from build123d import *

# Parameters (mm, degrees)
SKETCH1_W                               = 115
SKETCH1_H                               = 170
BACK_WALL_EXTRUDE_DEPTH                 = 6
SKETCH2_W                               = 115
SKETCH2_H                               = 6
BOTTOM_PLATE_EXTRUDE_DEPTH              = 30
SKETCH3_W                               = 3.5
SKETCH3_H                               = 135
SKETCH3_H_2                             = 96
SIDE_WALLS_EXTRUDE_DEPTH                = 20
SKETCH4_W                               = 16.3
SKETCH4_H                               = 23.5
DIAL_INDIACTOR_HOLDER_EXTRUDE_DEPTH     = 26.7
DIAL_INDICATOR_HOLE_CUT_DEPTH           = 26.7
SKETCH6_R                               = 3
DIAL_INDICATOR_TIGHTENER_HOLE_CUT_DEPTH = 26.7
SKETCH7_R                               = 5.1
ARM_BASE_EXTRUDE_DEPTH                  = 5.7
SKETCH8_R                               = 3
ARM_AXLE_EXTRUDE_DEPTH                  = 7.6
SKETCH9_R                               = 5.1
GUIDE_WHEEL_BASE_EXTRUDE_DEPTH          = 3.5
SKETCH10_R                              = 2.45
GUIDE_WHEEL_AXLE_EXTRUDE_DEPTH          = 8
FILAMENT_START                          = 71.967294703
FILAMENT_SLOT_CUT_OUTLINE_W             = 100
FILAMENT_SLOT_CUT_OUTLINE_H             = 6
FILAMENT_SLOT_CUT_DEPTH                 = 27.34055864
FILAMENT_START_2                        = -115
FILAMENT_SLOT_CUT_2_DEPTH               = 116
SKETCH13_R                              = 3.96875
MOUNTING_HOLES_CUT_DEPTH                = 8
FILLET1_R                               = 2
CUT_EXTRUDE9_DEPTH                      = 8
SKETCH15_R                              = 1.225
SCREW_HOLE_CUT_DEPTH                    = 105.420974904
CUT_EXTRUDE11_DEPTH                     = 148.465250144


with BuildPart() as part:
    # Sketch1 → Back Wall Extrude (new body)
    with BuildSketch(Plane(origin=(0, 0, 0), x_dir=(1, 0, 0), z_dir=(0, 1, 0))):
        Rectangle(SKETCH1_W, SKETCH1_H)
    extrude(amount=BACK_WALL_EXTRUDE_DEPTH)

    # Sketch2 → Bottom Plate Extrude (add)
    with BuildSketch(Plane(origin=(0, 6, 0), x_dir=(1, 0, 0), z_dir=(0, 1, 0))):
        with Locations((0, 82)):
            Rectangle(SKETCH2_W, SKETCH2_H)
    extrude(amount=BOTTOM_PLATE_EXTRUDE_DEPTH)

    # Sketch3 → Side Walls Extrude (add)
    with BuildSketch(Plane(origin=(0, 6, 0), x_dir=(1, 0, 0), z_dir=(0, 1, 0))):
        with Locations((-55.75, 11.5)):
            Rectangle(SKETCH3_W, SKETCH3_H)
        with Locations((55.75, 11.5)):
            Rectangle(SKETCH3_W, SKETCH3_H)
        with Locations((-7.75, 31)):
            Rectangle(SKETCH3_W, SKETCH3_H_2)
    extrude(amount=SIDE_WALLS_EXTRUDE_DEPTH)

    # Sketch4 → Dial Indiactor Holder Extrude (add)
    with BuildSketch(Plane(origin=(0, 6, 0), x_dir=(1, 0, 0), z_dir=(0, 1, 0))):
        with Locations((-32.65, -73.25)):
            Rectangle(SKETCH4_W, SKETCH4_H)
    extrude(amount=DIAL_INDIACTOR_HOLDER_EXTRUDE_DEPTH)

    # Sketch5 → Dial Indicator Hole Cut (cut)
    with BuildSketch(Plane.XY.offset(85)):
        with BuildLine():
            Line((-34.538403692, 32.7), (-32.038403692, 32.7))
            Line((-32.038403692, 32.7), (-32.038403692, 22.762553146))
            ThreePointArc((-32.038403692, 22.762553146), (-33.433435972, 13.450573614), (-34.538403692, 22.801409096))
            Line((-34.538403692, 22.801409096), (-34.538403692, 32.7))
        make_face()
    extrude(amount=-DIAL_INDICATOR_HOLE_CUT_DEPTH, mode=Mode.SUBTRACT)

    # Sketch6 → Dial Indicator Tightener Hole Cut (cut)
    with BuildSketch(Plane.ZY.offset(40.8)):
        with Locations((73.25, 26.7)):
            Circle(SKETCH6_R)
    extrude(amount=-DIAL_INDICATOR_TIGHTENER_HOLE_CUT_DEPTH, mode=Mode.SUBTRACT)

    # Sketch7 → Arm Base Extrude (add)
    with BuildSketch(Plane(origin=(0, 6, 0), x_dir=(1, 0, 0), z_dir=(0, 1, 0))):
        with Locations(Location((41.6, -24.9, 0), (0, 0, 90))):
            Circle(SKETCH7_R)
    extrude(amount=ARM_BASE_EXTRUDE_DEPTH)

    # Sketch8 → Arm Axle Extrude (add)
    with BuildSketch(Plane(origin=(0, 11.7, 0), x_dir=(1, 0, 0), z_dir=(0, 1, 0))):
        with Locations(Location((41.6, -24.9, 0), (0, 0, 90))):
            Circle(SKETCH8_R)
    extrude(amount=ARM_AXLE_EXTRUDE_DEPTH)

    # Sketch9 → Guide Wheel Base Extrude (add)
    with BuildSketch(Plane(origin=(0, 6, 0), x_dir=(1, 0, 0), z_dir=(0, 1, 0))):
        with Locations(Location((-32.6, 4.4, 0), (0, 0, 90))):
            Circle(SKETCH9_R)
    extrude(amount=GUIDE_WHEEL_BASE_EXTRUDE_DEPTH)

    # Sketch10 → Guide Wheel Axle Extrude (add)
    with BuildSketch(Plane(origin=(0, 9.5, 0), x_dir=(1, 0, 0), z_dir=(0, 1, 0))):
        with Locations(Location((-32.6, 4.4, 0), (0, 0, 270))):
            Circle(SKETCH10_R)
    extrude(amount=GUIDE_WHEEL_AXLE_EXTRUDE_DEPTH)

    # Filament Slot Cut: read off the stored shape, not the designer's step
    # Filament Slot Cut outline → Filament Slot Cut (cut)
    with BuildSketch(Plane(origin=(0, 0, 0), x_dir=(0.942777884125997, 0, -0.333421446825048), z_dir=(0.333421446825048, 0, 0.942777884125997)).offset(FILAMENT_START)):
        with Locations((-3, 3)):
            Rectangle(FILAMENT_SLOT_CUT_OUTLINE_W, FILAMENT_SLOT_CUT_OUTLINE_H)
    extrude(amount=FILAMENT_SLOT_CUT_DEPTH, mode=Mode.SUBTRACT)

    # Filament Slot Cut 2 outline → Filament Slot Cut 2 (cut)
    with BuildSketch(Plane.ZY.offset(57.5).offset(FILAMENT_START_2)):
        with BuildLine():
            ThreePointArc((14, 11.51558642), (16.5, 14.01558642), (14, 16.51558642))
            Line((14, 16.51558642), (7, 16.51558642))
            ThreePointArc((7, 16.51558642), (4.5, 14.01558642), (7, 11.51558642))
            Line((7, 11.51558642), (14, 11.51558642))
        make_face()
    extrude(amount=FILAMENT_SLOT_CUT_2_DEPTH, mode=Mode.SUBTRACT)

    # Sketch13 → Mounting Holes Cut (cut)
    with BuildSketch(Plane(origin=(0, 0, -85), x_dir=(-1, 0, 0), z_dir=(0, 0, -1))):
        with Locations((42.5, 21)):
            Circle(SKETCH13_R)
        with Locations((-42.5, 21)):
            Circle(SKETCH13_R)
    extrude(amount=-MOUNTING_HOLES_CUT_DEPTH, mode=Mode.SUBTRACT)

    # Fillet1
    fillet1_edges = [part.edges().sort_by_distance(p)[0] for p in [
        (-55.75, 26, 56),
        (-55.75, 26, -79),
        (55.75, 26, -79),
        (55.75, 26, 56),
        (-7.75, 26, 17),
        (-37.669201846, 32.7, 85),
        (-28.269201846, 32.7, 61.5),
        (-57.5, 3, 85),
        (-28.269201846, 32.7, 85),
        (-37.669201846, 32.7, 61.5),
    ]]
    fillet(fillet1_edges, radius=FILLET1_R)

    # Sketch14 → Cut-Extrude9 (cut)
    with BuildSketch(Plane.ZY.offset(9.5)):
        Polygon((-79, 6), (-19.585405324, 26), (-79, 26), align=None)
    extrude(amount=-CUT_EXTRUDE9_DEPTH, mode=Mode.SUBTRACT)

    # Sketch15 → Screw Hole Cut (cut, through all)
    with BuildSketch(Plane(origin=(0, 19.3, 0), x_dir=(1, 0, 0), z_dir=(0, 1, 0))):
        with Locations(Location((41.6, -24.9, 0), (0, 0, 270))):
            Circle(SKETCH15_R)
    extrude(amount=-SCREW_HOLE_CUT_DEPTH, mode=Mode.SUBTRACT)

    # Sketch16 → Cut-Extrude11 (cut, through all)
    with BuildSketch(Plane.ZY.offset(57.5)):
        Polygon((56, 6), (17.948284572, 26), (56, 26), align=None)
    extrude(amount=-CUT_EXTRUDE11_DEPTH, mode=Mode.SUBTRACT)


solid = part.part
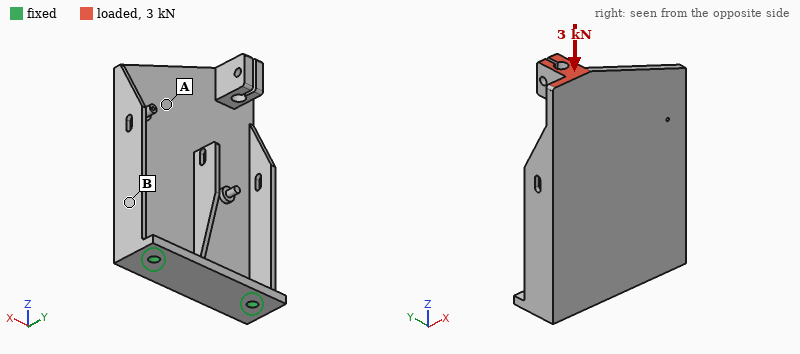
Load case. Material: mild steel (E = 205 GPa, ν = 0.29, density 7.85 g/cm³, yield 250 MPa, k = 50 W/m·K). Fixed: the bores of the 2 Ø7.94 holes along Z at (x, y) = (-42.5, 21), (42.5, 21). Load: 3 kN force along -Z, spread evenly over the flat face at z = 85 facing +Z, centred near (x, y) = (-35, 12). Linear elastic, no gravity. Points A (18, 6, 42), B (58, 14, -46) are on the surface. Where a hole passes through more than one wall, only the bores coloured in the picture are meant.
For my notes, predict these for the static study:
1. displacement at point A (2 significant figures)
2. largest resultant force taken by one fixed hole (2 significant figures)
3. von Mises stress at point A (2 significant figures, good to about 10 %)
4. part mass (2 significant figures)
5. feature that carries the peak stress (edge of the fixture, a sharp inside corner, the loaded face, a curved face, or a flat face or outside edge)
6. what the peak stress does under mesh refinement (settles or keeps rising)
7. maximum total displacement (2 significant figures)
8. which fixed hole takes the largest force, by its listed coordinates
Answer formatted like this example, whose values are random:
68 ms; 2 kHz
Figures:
0.028 mm; 2.6 kN; 23 MPa; 1.2 kg; edge of the fixture; keeps rising; 0.17 mm; (-42.5, 21)
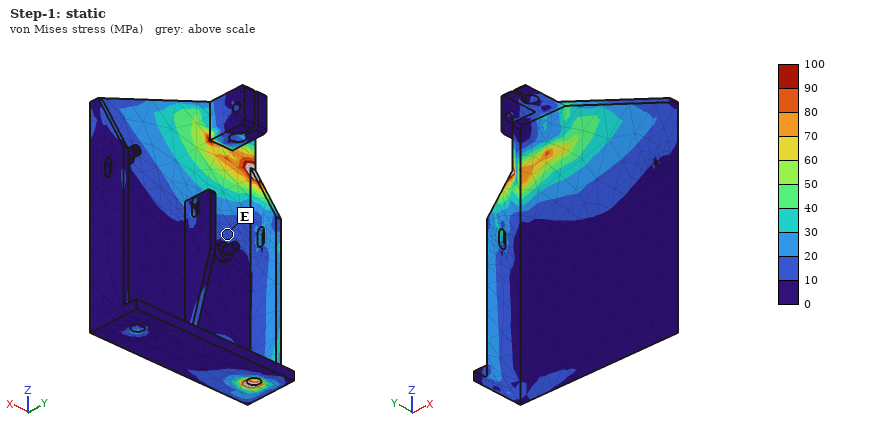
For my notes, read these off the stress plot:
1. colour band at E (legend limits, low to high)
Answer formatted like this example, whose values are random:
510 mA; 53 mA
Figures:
10 to 20 MPa
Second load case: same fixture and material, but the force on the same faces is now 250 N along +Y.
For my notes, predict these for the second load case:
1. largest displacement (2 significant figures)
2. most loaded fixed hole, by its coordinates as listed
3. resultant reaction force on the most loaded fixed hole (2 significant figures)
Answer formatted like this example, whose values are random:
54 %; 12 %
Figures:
0.34 mm; (-42.5, 21); 230 N
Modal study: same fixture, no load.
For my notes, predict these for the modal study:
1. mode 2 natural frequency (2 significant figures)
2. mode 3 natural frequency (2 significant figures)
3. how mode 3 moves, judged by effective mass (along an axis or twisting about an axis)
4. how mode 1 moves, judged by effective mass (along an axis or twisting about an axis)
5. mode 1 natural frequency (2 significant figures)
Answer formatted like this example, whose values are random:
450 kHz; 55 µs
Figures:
600 Hz; 1400 Hz; along X; along Y; 290 Hz
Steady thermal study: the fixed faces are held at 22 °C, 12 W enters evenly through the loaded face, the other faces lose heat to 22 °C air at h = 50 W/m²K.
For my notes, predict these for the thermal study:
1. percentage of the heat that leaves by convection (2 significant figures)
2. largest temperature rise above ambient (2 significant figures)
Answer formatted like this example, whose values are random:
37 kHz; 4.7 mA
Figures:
96 %; 26 K
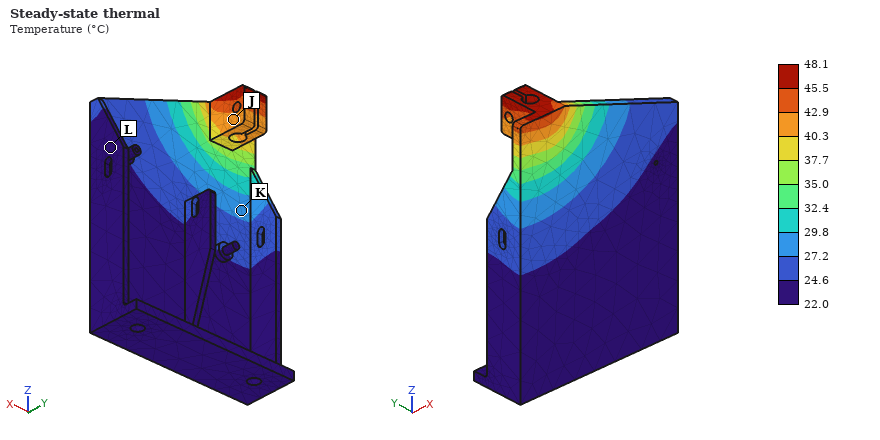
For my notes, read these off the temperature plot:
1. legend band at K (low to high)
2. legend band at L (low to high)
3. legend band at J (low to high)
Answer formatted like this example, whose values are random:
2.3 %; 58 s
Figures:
27.2 to 29.8 °C; 22.0 to 24.6 °C; 40.3 to 42.9 °C
